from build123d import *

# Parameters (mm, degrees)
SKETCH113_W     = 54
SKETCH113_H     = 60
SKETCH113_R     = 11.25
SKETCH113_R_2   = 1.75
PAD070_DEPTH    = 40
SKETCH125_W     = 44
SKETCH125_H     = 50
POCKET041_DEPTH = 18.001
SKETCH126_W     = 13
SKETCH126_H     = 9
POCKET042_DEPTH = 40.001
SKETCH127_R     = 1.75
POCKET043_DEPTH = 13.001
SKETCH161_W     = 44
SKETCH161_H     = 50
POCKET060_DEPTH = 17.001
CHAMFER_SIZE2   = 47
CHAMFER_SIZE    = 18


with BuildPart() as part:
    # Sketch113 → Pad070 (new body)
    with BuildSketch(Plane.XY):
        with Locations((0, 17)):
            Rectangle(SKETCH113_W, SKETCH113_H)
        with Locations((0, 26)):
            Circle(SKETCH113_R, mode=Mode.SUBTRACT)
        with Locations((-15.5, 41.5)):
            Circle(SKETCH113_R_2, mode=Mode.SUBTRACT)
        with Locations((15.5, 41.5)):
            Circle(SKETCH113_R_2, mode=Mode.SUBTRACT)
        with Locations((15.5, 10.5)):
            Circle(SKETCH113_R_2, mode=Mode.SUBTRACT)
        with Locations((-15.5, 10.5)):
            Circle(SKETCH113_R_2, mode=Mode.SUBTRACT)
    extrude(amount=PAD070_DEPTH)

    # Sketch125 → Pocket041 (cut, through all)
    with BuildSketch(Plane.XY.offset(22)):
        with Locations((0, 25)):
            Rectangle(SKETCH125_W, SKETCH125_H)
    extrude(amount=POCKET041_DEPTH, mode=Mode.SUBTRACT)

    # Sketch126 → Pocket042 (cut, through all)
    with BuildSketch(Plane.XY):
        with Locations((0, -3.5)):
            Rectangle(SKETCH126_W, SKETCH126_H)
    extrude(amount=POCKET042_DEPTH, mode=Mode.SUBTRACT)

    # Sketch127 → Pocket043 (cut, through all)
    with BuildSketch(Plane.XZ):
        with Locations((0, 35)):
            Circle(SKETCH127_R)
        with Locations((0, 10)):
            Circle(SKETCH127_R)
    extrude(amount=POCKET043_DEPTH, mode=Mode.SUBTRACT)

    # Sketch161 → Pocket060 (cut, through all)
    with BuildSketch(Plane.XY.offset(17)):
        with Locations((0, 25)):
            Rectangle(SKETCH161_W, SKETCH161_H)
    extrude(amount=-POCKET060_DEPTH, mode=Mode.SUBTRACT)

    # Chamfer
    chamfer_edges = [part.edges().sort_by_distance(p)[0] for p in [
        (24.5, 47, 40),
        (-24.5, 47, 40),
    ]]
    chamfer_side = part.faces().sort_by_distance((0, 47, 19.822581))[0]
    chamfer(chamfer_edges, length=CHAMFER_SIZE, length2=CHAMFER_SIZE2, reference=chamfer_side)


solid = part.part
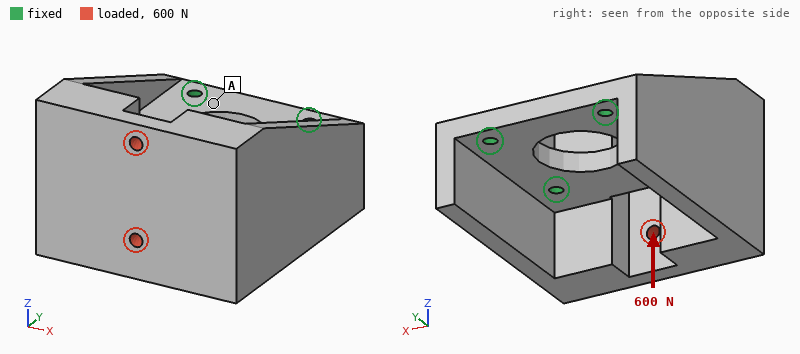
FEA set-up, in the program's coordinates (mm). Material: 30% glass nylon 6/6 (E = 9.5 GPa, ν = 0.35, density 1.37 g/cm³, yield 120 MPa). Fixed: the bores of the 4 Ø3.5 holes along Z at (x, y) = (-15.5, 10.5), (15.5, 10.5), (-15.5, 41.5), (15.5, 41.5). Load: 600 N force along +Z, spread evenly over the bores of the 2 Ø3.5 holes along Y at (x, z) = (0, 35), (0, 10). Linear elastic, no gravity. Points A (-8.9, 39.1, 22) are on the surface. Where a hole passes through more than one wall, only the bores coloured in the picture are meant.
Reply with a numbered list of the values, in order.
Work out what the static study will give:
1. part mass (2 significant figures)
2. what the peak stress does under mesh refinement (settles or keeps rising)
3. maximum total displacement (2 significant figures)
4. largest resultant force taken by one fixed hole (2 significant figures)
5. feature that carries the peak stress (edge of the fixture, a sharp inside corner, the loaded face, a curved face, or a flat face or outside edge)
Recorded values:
1. 64 g
2. keeps rising
3. 99 µm
4. 460 N
5. edge of the fixture
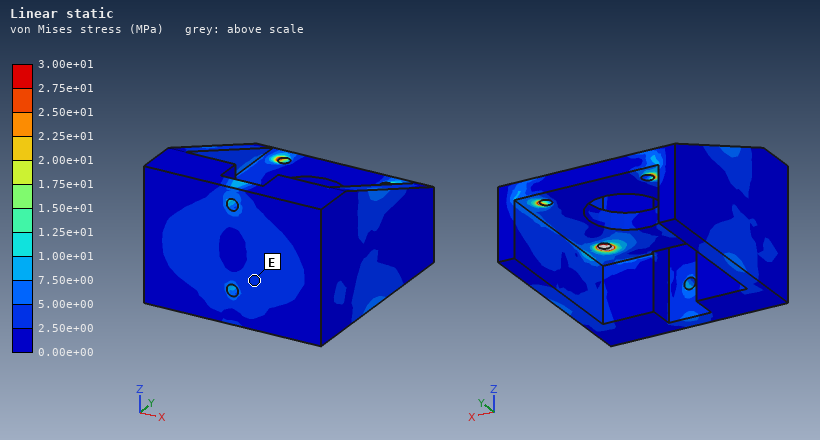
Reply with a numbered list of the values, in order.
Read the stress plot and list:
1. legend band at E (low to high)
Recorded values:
1. 2.50e+00 to 5.00e+00 MPa
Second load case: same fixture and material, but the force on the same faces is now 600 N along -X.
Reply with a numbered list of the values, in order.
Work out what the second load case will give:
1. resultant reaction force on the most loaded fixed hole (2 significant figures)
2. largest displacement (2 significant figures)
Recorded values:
1. 400 N
2. 35 µm
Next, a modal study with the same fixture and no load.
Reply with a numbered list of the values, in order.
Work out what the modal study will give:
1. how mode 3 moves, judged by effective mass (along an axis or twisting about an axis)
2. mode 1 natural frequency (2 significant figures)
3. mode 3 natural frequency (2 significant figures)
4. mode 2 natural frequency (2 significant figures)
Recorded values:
1. along Z
2. 2500 Hz
3. 4000 Hz
4. 2600 Hz
